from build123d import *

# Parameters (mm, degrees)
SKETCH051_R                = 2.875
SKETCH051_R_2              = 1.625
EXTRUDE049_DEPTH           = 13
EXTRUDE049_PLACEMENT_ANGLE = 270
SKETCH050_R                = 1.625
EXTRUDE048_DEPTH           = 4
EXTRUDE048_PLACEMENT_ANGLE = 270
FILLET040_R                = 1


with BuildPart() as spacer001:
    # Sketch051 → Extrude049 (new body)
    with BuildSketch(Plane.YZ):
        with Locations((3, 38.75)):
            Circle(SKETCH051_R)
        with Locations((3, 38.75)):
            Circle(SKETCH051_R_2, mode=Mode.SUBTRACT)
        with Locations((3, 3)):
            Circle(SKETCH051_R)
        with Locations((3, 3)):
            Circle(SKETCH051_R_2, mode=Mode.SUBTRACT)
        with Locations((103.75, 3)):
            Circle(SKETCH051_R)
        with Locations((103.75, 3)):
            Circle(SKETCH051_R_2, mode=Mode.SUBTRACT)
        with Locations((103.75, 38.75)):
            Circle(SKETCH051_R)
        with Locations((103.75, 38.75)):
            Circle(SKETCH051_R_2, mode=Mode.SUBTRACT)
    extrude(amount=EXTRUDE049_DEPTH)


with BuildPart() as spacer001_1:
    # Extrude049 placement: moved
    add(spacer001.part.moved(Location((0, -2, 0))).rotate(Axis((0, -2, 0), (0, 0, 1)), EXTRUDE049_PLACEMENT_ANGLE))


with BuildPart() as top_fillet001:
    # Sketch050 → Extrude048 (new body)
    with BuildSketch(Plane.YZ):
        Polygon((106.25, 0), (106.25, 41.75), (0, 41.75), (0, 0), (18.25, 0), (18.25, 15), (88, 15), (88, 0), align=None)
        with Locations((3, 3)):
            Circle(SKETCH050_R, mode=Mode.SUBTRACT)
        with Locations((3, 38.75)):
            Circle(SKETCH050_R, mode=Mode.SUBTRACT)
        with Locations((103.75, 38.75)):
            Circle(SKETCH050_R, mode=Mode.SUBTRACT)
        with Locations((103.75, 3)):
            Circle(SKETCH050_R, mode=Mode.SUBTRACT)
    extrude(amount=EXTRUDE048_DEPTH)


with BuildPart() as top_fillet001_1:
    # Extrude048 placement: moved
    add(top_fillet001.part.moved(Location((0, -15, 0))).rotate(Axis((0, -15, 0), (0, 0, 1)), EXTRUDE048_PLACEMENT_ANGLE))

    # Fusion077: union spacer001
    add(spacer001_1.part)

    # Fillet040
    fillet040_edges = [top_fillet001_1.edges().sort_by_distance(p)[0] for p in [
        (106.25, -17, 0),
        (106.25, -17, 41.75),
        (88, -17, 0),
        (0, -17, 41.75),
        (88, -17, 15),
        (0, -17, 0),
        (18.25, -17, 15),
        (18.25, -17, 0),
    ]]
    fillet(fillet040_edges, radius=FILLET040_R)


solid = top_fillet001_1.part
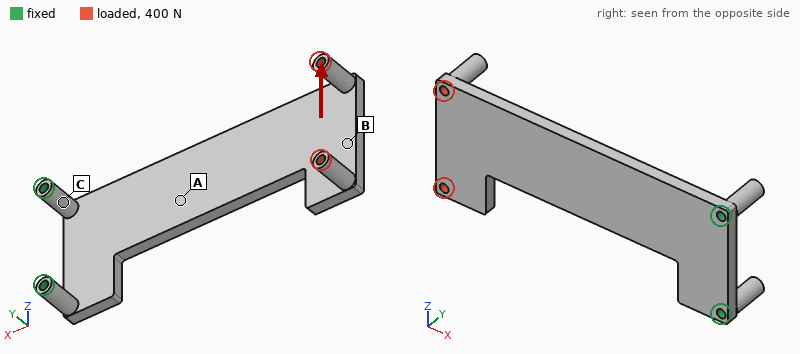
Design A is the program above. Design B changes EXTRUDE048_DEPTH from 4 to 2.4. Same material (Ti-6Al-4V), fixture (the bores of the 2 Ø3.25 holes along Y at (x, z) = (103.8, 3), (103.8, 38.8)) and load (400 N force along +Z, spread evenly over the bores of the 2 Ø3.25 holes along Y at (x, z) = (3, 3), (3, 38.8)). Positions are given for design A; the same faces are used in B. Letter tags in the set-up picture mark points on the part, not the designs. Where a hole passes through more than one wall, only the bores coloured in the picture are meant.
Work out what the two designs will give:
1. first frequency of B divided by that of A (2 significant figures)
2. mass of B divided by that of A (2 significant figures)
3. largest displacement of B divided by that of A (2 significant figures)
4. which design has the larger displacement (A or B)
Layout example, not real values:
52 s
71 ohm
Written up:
0.59
0.63
3.5
B
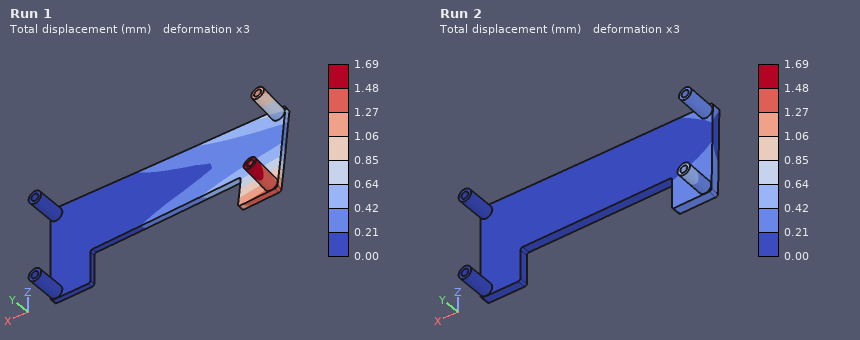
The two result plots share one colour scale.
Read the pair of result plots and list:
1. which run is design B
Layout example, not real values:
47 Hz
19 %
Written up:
Run 1
